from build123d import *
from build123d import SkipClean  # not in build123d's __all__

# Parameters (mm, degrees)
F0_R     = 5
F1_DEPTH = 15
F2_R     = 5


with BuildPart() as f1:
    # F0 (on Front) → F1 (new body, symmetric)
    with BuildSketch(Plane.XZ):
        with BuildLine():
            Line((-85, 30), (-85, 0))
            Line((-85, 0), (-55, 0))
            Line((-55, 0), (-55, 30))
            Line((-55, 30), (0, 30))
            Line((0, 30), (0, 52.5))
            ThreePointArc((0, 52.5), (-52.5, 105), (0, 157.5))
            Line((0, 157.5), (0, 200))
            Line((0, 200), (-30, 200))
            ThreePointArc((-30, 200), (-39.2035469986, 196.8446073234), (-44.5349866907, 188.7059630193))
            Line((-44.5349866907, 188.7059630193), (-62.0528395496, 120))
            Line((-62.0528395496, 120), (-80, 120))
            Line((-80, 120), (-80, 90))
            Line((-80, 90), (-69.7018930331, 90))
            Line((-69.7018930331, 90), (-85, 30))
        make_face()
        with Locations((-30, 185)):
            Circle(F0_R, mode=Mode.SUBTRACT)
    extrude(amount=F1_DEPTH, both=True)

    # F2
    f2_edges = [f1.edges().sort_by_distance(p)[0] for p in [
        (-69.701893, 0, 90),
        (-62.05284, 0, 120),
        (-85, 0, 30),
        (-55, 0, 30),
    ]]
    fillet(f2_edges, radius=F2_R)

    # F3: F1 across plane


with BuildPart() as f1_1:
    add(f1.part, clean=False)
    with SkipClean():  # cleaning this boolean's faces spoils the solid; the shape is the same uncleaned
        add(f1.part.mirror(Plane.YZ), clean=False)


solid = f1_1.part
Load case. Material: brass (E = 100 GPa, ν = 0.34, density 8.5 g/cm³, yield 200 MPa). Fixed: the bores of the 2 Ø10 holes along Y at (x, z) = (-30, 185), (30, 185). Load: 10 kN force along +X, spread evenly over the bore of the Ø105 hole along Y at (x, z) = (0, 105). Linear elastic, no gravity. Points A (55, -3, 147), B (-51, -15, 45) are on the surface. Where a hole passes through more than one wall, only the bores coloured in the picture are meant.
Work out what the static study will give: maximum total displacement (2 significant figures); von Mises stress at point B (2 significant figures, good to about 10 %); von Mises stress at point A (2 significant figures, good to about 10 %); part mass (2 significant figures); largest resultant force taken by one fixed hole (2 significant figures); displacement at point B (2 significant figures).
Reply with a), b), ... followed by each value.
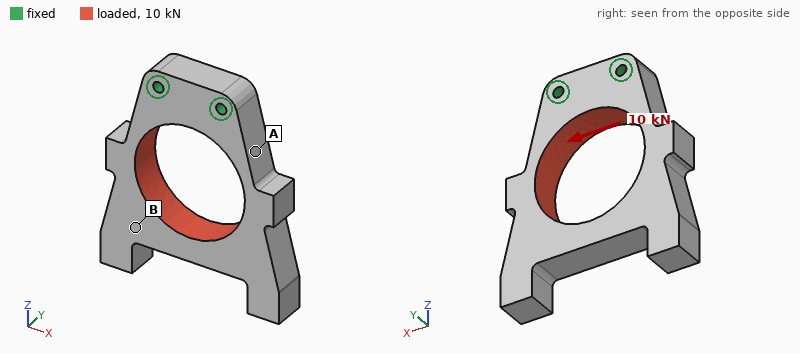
a) 0.27 mm
b) 8.3 MPa
c) 58 MPa
d) 3.9 kg
e) 12 kN
f) 0.22 mm
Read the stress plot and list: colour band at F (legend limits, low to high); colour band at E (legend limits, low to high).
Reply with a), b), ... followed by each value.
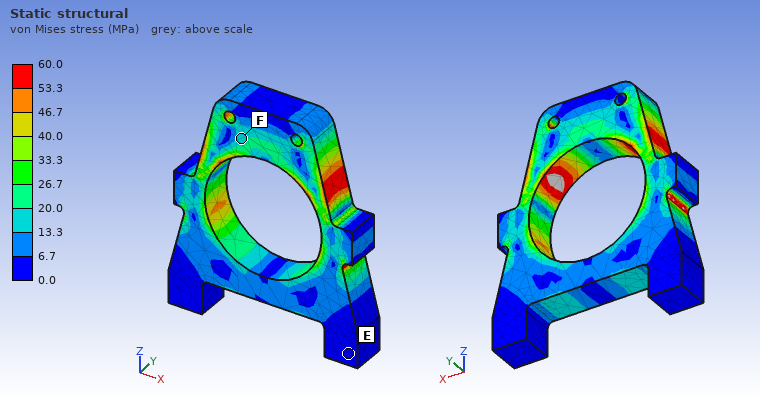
a) 13.3 to 20.0 MPa
b) 0.0 to 6.7 MPa
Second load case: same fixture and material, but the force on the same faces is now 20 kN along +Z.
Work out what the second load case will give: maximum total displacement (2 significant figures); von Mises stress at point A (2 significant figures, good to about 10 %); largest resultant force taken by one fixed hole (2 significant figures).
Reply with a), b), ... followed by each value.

a) 62 µm
b) 31 MPa
c) 11 kN
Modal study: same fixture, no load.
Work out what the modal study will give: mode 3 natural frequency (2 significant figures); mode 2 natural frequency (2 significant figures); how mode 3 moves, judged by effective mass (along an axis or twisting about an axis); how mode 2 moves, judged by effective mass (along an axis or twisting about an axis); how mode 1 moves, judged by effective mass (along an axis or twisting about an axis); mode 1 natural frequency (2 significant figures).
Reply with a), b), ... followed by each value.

a) 590 Hz
b) 500 Hz
c) twisting about Z
d) along X
e) along Y
f) 300 Hz
